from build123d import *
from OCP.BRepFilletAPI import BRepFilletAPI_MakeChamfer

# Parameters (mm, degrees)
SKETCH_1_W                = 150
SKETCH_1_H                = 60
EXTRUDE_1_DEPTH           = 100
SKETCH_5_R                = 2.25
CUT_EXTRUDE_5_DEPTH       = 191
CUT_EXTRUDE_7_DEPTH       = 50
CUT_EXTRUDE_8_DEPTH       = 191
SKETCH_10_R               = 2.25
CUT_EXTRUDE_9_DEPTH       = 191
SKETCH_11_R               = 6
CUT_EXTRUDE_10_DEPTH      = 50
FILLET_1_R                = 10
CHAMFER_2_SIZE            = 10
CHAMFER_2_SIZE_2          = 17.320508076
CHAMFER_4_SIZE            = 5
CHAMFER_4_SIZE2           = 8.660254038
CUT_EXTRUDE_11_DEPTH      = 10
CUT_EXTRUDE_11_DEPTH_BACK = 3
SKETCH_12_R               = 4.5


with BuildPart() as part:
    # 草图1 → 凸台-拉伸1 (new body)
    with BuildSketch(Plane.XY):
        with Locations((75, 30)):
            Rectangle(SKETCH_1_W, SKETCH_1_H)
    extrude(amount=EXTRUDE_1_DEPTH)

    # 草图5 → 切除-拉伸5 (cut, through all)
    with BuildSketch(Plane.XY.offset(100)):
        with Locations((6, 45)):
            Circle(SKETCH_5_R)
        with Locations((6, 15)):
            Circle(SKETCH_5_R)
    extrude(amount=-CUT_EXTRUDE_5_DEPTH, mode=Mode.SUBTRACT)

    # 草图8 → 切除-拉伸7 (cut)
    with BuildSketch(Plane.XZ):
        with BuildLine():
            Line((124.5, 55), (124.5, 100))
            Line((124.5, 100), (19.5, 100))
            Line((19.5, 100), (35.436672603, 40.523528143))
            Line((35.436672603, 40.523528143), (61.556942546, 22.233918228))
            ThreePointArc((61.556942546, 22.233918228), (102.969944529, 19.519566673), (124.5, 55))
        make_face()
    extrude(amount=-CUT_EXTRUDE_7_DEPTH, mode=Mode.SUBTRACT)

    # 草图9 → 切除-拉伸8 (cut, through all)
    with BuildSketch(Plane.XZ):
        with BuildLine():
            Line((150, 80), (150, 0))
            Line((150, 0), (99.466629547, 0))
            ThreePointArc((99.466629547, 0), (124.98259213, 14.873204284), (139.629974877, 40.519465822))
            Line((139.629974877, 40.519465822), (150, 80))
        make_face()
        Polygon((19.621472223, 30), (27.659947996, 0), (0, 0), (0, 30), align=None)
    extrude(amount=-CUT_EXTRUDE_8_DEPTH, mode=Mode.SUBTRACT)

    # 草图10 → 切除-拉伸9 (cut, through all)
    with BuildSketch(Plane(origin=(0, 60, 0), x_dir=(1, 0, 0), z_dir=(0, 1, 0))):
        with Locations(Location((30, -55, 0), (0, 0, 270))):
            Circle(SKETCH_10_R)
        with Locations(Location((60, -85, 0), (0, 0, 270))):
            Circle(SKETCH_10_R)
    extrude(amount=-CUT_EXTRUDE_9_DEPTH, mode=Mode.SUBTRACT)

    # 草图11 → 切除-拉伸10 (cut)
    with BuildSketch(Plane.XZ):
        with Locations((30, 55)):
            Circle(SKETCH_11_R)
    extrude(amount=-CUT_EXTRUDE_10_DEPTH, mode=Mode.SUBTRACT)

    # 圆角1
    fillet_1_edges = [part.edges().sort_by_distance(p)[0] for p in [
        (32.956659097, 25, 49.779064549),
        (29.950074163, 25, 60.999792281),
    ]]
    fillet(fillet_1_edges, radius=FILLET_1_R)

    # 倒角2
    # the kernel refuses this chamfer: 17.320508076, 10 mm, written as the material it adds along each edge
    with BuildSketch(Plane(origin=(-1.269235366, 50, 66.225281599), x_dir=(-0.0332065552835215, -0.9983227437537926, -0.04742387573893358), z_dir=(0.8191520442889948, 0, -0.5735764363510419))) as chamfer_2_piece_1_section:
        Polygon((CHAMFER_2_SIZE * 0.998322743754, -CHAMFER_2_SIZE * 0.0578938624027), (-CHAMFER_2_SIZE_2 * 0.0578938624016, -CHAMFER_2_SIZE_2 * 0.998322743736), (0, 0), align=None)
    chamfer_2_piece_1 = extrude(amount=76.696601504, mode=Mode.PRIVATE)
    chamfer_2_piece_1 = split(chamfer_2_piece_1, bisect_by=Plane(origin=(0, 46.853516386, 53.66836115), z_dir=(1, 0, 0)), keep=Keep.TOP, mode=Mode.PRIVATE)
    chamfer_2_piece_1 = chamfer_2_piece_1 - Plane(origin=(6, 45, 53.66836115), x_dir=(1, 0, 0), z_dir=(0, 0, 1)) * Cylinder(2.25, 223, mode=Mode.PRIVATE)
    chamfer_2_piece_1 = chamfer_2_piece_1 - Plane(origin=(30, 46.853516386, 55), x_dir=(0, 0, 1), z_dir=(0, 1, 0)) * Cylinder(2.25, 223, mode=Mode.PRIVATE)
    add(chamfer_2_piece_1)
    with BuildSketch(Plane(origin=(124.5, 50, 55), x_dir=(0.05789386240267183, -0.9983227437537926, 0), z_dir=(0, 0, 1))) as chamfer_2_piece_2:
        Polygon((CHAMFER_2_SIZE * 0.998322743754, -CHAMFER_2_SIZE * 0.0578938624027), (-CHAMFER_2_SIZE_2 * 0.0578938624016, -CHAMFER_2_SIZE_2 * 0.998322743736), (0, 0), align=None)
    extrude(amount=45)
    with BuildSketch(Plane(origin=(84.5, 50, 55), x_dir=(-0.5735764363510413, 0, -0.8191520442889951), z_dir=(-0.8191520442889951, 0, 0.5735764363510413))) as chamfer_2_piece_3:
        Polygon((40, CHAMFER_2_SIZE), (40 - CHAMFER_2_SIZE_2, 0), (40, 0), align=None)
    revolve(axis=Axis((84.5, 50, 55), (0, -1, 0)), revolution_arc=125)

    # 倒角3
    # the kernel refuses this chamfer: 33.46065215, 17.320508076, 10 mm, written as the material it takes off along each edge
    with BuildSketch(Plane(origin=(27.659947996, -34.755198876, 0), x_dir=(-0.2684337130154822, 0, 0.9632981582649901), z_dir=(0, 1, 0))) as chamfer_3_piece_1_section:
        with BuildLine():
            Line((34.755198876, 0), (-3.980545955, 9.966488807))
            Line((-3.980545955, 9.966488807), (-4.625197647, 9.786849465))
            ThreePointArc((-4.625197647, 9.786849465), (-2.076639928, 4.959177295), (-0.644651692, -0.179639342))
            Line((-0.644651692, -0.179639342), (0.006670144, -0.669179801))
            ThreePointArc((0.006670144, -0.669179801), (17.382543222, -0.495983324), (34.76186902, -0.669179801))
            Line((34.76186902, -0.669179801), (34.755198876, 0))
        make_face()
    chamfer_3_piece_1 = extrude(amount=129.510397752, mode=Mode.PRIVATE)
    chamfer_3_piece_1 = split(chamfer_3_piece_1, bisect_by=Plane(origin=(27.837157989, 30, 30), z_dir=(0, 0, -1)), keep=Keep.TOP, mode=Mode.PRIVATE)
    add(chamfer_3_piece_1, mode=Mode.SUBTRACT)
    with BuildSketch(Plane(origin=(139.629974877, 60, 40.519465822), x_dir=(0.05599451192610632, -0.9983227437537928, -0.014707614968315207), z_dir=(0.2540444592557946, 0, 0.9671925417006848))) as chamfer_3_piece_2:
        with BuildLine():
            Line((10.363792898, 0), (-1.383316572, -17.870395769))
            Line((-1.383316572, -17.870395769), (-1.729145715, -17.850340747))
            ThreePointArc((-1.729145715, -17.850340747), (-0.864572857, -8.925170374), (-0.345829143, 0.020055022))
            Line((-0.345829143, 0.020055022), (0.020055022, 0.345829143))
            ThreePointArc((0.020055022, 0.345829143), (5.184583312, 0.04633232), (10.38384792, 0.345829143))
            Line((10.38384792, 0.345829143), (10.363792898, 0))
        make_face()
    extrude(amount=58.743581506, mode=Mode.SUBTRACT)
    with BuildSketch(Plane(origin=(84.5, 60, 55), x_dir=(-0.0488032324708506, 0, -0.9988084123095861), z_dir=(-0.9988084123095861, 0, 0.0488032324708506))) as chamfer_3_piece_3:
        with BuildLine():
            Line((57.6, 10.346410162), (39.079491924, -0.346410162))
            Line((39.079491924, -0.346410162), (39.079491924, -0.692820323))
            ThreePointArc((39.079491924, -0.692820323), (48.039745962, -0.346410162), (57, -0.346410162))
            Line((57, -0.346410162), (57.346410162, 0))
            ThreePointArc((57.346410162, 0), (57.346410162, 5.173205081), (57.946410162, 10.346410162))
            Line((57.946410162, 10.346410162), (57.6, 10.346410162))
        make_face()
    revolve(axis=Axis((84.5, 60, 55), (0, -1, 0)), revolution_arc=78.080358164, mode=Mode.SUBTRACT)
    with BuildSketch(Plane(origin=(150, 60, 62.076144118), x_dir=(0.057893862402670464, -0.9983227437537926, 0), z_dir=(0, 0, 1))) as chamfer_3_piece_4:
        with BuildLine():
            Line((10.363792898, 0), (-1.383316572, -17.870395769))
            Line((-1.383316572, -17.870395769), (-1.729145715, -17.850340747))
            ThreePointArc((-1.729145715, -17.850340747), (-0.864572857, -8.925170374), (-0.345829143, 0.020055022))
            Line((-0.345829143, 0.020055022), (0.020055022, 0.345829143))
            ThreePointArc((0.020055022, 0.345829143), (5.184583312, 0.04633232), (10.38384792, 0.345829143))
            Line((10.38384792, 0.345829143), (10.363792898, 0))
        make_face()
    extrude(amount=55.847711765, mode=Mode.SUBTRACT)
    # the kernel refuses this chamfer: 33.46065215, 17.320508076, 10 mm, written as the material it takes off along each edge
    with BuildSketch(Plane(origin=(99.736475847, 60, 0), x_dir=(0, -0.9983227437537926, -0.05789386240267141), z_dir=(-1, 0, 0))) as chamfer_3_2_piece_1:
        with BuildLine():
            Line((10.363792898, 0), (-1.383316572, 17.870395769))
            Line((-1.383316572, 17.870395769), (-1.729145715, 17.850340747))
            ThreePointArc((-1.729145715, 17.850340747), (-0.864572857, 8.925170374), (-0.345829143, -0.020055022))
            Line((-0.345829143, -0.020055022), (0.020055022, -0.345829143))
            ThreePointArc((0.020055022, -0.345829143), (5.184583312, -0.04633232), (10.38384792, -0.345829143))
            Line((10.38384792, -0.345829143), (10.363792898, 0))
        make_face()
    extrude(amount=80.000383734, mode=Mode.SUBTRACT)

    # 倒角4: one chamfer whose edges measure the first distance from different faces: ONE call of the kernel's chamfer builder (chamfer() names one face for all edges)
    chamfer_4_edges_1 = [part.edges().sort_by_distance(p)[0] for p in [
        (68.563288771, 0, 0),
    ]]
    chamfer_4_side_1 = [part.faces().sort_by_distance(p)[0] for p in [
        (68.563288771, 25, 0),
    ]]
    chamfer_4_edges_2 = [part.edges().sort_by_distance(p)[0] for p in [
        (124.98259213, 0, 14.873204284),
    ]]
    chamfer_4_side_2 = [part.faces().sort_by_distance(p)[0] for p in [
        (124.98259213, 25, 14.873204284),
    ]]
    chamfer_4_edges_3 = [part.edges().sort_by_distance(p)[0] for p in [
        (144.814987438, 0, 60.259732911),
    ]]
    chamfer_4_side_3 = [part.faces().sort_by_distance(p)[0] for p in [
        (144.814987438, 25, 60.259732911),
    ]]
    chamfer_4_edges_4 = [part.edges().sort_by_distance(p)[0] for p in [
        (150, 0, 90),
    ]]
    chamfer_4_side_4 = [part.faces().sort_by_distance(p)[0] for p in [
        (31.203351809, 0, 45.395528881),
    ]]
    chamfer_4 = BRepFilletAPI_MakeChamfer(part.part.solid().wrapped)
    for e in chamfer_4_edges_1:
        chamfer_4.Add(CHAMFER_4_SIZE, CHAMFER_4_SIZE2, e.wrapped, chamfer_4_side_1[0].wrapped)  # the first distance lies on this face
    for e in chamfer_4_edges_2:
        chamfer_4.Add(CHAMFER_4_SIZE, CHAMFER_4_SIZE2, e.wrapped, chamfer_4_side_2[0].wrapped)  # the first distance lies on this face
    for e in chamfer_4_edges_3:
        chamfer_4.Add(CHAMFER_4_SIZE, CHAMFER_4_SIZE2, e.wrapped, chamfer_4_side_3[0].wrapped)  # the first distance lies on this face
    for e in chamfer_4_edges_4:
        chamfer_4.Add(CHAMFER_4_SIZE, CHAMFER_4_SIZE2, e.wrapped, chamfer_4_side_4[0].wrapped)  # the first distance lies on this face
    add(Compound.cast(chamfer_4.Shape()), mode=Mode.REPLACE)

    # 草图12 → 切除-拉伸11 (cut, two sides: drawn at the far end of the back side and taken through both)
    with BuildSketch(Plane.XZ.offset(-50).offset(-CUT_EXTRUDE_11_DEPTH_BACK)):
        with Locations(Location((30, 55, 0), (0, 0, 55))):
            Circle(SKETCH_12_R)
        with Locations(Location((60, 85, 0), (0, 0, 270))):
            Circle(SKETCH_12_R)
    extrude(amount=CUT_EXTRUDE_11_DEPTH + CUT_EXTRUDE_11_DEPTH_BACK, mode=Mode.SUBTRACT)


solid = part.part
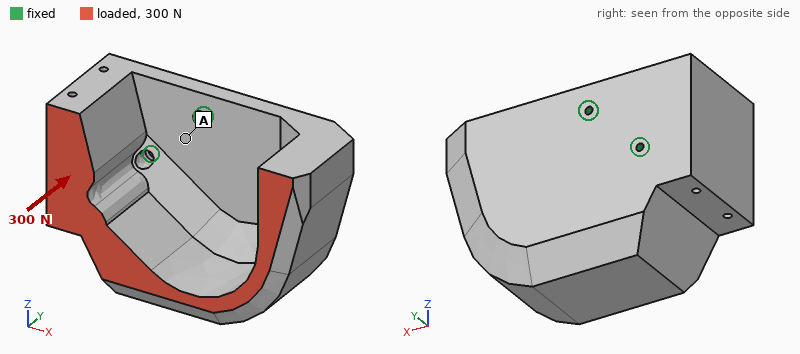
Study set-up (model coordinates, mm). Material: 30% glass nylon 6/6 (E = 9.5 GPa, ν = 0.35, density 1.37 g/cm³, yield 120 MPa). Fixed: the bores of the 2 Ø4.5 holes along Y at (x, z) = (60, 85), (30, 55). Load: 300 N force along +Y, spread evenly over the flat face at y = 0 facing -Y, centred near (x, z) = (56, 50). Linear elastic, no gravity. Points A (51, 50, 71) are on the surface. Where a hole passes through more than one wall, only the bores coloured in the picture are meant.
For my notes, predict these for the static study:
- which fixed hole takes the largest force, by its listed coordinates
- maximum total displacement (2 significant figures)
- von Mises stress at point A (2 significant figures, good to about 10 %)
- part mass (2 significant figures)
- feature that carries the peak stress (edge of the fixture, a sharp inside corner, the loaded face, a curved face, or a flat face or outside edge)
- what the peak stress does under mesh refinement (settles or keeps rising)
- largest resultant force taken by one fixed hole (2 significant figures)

(30, 55)
0.23 mm
1.3 MPa
560 g
edge of the fixture
keeps rising
200 N
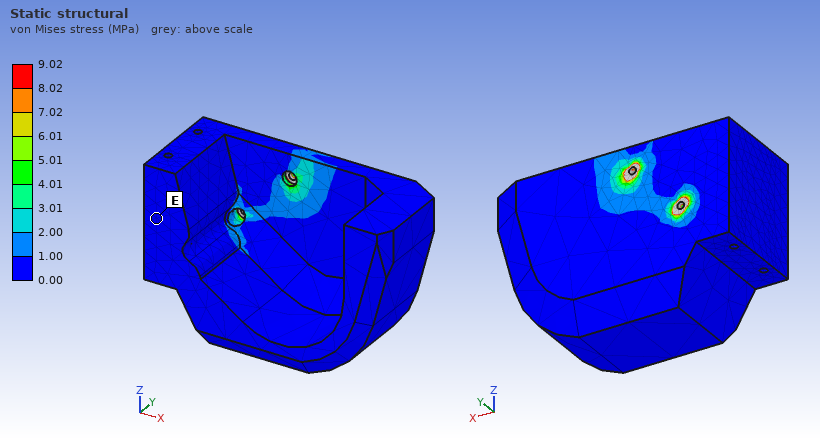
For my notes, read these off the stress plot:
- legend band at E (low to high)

0.00 to 1.00 MPa
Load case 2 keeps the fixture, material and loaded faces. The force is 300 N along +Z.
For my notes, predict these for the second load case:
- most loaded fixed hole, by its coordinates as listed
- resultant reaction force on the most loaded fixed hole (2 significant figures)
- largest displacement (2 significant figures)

(60, 85)
340 N
0.42 mm
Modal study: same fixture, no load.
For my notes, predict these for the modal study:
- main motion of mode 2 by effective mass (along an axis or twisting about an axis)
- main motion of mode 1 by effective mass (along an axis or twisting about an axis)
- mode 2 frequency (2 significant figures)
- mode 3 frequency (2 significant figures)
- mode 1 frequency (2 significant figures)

along Z
along Y
500 Hz
900 Hz
200 Hz
